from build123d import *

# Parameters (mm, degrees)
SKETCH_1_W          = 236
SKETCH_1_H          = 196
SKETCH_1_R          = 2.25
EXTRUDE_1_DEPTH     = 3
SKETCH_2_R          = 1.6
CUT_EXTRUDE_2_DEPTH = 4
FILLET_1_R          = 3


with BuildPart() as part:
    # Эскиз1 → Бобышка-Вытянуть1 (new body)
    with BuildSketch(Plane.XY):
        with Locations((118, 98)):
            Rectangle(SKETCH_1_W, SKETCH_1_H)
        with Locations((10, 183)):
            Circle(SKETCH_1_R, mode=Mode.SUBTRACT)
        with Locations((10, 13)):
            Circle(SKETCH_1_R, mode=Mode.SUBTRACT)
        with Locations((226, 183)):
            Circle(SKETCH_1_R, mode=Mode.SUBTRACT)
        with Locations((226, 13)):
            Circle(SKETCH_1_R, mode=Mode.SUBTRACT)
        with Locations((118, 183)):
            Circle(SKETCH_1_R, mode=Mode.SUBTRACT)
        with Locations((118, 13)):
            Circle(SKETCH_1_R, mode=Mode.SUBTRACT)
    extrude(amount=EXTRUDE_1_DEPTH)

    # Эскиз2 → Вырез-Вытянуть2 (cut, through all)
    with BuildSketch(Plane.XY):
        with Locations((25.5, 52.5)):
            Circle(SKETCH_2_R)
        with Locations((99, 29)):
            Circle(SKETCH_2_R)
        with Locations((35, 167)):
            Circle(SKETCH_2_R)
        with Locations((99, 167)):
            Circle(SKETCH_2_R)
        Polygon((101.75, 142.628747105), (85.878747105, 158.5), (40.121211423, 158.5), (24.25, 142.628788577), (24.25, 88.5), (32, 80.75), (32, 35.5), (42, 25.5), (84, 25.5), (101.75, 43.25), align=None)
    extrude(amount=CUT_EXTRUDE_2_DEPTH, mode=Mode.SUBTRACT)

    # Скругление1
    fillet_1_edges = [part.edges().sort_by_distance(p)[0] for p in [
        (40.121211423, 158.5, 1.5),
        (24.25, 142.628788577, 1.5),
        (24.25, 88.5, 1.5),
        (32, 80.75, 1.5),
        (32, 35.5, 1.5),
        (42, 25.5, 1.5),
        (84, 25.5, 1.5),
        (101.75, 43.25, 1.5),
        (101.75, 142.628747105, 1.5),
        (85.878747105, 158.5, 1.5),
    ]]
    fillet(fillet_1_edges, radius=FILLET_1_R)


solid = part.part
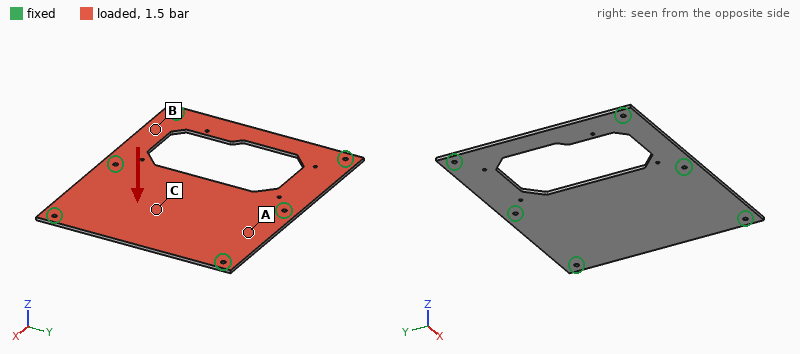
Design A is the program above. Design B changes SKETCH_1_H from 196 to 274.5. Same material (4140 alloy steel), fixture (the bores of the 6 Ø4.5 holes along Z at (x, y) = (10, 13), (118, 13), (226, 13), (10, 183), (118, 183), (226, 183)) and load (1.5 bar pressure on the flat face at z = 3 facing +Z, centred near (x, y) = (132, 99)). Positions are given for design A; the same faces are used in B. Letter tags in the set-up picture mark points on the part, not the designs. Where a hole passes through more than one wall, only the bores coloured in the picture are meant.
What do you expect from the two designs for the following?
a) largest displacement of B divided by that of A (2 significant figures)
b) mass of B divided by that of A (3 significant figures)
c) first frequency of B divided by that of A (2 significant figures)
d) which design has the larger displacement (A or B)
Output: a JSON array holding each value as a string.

["0.82", "1.50", "0.98", "A"]
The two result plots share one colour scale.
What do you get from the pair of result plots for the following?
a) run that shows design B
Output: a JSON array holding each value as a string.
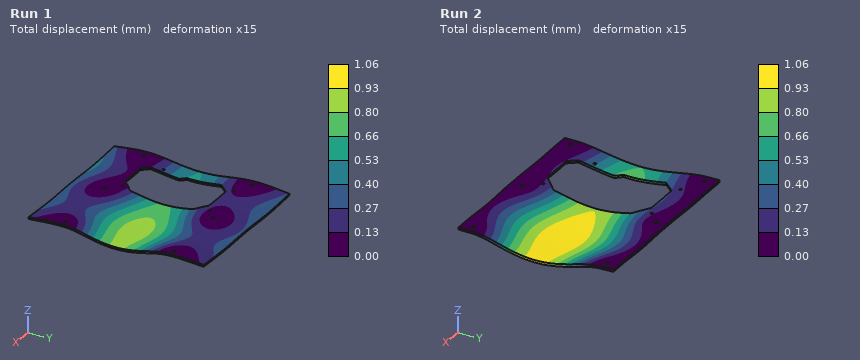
["Run 1"]
